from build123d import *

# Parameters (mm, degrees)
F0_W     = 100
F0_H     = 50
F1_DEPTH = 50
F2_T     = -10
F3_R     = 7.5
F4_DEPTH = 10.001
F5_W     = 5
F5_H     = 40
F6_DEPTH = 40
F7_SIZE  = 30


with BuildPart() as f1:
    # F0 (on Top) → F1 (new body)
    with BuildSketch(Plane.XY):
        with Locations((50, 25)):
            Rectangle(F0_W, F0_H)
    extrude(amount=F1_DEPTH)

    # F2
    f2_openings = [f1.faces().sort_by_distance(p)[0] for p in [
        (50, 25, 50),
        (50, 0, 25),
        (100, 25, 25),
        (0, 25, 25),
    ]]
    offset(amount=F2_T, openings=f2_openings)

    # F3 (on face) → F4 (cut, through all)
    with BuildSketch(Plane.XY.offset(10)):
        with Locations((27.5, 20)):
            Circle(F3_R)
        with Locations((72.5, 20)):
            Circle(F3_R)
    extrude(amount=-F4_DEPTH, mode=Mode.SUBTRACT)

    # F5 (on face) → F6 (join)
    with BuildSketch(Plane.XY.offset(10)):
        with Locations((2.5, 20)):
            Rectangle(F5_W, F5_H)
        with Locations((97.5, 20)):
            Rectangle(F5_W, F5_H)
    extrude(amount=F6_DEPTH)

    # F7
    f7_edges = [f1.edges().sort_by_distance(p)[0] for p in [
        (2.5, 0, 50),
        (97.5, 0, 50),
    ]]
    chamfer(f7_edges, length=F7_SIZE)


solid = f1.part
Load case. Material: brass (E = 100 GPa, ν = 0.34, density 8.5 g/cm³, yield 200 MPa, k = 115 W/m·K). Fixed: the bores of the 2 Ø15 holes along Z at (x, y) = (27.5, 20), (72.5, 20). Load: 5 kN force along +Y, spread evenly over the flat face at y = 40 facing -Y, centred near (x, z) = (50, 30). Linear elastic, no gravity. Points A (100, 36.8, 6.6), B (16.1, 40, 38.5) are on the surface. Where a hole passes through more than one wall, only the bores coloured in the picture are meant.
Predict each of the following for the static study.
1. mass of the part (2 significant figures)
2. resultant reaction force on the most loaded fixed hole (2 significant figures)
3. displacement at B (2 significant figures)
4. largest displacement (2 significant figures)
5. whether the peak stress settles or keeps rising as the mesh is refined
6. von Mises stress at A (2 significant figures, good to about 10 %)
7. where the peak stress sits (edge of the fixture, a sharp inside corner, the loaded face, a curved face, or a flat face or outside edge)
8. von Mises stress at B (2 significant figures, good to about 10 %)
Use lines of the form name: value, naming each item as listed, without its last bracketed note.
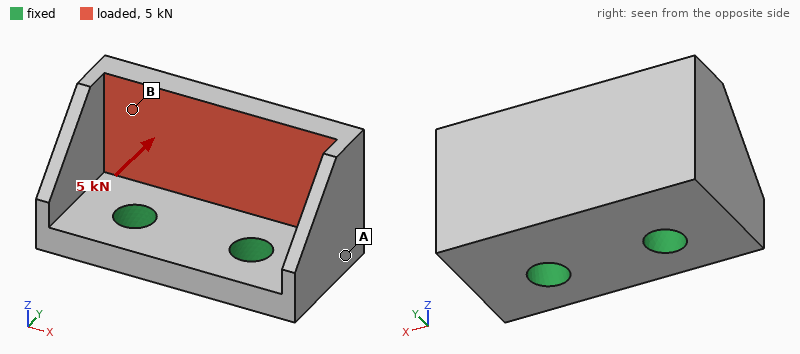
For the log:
mass of the part: 830 g
resultant reaction force on the most loaded fixed hole: 2.5 kN
displacement at B: 0.065 mm
largest displacement: 0.12 mm
whether the peak stress settles or keeps rising as the mesh is refined: keeps rising
von Mises stress at A: 9.7 MPa
where the peak stress sits: edge of the fixture
von Mises stress at B: 25 MPa
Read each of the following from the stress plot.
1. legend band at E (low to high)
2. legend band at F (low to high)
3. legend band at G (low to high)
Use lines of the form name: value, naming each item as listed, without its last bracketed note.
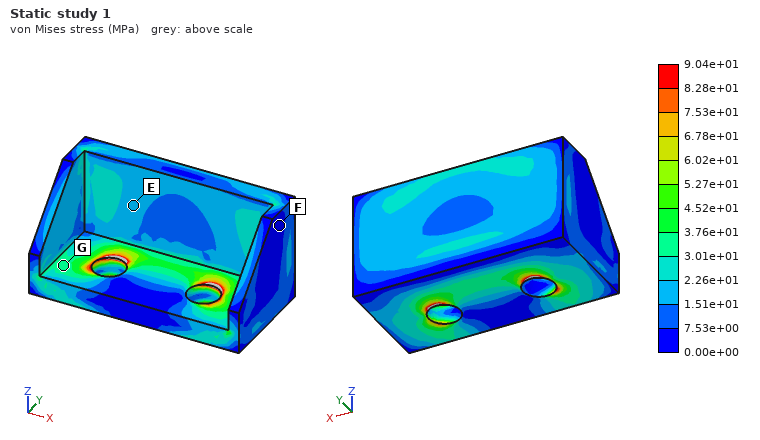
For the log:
legend band at E: 1.51e+01 to 2.26e+01 MPa
legend band at F: 0.00e+00 to 7.53e+00 MPa
legend band at G: 3.01e+01 to 3.76e+01 MPa
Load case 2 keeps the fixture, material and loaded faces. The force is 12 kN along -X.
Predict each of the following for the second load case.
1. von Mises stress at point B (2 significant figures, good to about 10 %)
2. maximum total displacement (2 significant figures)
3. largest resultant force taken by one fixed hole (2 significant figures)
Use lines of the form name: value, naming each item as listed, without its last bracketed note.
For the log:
von Mises stress at point B: 27 MPa
maximum total displacement: 0.12 mm
largest resultant force taken by one fixed hole: 8.5 kN
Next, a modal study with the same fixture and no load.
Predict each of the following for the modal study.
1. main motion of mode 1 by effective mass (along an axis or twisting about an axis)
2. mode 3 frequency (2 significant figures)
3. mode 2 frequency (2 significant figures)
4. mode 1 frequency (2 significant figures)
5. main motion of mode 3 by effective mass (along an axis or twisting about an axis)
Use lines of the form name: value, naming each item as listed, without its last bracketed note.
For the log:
main motion of mode 1 by effective mass: along Y
mode 3 frequency: 4300 Hz
mode 2 frequency: 2500 Hz
mode 1 frequency: 2000 Hz
main motion of mode 3 by effective mass: along X
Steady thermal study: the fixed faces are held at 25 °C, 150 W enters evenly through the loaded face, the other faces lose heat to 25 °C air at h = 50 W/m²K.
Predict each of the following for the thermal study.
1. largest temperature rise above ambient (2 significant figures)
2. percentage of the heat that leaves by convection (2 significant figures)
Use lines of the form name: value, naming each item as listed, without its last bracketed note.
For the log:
largest temperature rise above ambient: 47 K
percentage of the heat that leaves by convection: 15 %
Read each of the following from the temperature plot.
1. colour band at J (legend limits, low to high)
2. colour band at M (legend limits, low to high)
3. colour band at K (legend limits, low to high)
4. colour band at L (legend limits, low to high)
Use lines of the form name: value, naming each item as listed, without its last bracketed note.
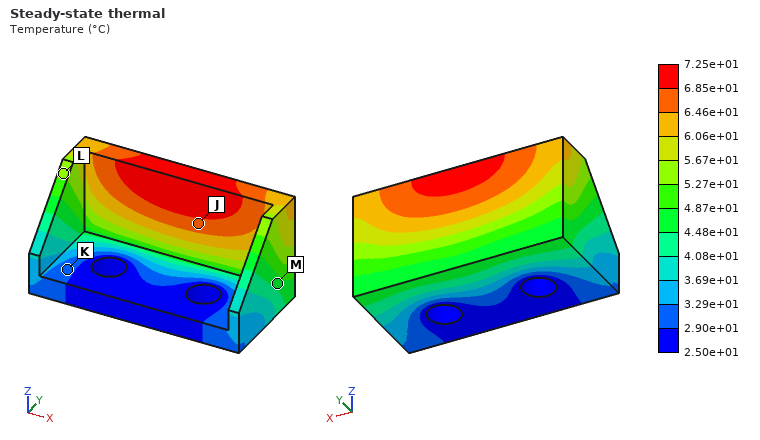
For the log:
colour band at J: 6.46e+01 to 6.85e+01 °C
colour band at M: 4.48e+01 to 4.87e+01 °C
colour band at K: 2.90e+01 to 3.29e+01 °C
colour band at L: 5.27e+01 to 5.67e+01 °C
